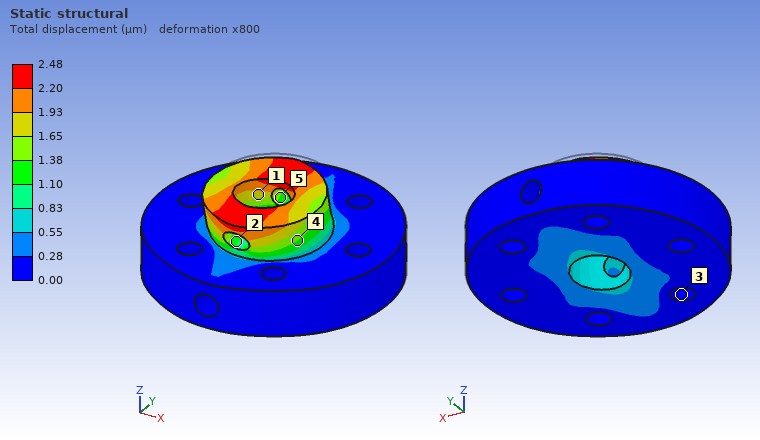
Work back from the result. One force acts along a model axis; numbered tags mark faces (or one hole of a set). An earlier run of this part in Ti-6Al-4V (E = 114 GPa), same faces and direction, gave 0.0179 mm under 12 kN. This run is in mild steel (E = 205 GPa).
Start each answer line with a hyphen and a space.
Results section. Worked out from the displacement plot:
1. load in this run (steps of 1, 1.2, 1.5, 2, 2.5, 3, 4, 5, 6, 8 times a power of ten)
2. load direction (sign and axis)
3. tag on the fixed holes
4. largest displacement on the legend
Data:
- 3 kN
- -Y
- 3
- 2.48 µm
